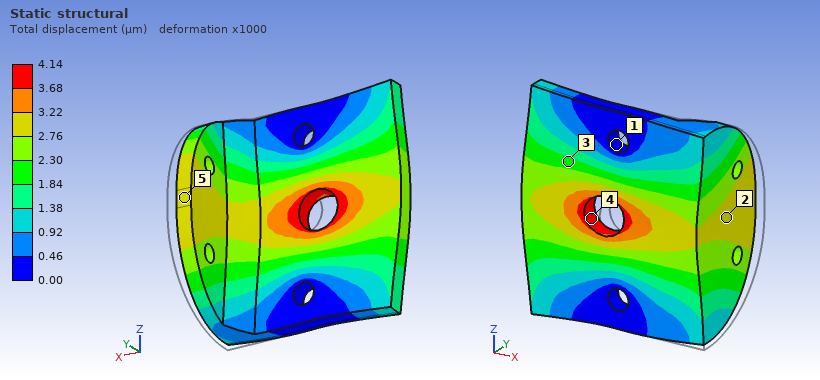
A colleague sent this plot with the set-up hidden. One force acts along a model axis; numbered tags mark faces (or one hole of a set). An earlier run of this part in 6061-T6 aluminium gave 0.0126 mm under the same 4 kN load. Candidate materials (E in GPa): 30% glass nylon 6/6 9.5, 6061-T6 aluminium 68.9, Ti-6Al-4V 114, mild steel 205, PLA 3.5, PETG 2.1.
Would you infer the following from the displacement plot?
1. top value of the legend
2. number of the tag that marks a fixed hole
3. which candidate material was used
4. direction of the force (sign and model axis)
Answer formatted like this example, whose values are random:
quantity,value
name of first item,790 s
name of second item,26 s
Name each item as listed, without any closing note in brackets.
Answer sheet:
quantity,value
top value of the legend,4.14 µm
number of the tag that marks a fixed hole,1
which candidate material was used,mild steel
direction of the force,-X
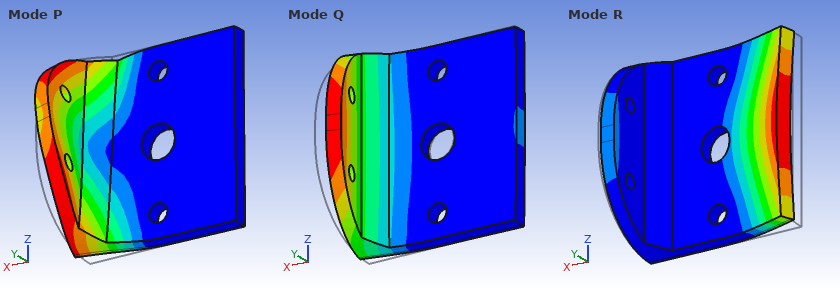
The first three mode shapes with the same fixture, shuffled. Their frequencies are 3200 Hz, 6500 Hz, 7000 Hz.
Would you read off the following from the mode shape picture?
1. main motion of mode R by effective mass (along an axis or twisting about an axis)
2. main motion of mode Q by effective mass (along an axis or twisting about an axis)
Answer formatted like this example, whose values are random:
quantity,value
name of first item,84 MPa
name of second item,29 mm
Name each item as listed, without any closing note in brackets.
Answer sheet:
quantity,value
main motion of mode R by effective mass,along Y
main motion of mode Q by effective mass,along Y
